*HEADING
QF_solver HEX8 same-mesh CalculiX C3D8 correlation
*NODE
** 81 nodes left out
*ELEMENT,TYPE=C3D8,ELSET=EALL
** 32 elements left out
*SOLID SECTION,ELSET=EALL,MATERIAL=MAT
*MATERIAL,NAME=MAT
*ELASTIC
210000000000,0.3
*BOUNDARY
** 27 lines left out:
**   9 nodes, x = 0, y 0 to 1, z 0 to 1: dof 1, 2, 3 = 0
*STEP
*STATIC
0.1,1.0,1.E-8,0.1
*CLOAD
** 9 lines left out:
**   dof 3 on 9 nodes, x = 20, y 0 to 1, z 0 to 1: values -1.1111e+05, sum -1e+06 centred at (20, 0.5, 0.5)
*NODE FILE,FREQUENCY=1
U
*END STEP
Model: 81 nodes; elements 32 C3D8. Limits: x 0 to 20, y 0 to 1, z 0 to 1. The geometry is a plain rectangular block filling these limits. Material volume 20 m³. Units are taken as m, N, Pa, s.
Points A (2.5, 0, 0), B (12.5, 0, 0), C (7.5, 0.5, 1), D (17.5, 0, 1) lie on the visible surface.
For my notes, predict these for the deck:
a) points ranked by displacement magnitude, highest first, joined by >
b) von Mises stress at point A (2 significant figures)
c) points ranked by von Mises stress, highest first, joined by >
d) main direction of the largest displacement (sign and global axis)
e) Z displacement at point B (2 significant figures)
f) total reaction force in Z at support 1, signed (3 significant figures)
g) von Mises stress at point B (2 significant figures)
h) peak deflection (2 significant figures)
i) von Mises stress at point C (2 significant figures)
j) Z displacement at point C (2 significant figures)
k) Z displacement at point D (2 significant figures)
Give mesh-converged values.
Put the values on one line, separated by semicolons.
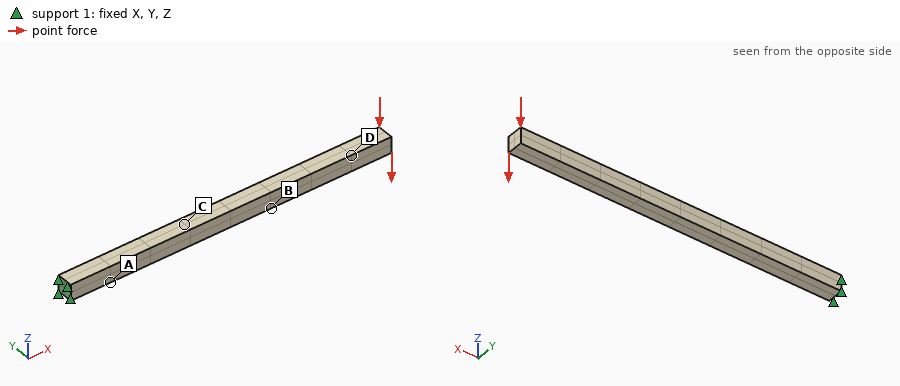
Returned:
D > B > C > A; 1.0e+08 Pa; A > C > B > D; -Z; -0.070 m; 1.00e+06 N; 4.5e+07 Pa; 0.15 m; 7.5e+07 Pa; -0.028 m; -0.12 m
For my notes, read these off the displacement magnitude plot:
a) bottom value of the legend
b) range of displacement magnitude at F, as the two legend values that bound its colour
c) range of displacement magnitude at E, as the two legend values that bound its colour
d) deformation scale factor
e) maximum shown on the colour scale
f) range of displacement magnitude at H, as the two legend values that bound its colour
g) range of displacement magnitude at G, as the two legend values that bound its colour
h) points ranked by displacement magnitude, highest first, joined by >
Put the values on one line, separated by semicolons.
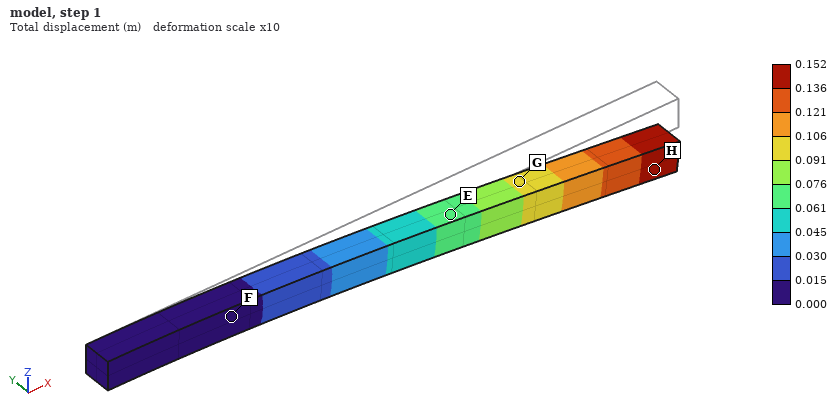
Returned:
0.000 m; 0.000 to 0.015 m; 0.061 to 0.076 m; 10; 0.152 m; 0.136 to 0.152 m; 0.091 to 0.106 m; H > G > E > F
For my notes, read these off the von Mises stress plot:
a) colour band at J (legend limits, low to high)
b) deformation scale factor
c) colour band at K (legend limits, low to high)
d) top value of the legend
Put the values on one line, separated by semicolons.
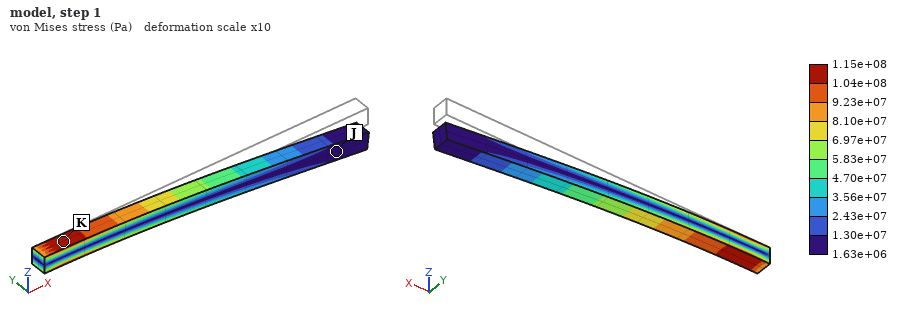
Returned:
1.63e+06 to 1.30e+07 Pa; 10; 1.04e+08 to 1.15e+08 Pa; 1.15e+08 Pa
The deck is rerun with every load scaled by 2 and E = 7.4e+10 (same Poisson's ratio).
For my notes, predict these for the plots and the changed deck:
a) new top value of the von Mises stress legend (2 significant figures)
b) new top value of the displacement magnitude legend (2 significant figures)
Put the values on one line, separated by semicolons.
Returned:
2.3e+08 Pa; 0.86 m
